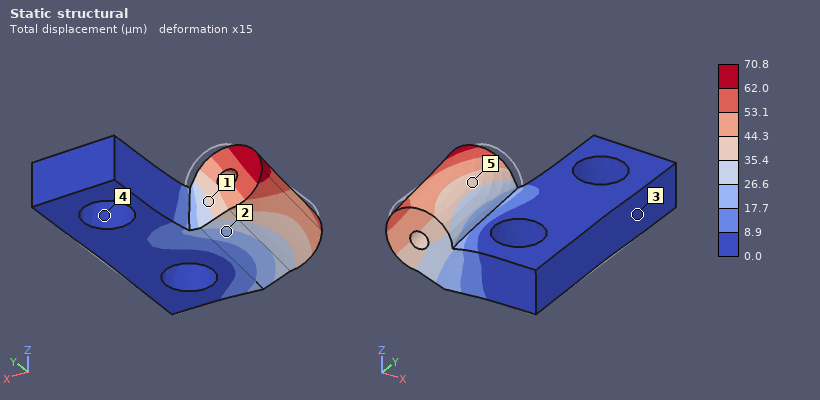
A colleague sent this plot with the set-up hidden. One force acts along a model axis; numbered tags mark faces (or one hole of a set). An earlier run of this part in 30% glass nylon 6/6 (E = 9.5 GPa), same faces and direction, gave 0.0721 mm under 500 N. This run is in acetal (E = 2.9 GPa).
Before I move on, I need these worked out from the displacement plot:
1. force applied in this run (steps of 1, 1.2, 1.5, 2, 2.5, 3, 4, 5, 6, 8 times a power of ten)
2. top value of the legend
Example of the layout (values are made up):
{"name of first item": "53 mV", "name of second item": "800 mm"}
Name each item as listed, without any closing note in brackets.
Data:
{"force applied in this run": "150 N", "top value of the legend": "70.8 µm"}
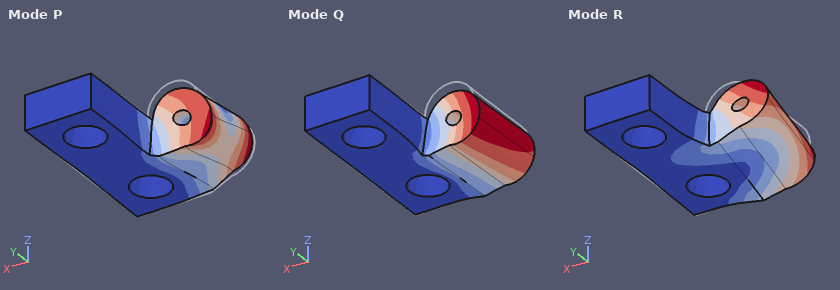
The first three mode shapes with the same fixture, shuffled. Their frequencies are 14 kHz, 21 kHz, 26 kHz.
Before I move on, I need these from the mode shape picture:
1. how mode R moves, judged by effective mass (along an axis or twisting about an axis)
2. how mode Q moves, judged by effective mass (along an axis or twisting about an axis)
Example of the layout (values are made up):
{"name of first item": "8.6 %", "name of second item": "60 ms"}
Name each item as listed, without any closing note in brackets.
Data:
{"how mode R moves, judged by effective mass": "along Y", "how mode Q moves, judged by effective mass": "along Z"}
